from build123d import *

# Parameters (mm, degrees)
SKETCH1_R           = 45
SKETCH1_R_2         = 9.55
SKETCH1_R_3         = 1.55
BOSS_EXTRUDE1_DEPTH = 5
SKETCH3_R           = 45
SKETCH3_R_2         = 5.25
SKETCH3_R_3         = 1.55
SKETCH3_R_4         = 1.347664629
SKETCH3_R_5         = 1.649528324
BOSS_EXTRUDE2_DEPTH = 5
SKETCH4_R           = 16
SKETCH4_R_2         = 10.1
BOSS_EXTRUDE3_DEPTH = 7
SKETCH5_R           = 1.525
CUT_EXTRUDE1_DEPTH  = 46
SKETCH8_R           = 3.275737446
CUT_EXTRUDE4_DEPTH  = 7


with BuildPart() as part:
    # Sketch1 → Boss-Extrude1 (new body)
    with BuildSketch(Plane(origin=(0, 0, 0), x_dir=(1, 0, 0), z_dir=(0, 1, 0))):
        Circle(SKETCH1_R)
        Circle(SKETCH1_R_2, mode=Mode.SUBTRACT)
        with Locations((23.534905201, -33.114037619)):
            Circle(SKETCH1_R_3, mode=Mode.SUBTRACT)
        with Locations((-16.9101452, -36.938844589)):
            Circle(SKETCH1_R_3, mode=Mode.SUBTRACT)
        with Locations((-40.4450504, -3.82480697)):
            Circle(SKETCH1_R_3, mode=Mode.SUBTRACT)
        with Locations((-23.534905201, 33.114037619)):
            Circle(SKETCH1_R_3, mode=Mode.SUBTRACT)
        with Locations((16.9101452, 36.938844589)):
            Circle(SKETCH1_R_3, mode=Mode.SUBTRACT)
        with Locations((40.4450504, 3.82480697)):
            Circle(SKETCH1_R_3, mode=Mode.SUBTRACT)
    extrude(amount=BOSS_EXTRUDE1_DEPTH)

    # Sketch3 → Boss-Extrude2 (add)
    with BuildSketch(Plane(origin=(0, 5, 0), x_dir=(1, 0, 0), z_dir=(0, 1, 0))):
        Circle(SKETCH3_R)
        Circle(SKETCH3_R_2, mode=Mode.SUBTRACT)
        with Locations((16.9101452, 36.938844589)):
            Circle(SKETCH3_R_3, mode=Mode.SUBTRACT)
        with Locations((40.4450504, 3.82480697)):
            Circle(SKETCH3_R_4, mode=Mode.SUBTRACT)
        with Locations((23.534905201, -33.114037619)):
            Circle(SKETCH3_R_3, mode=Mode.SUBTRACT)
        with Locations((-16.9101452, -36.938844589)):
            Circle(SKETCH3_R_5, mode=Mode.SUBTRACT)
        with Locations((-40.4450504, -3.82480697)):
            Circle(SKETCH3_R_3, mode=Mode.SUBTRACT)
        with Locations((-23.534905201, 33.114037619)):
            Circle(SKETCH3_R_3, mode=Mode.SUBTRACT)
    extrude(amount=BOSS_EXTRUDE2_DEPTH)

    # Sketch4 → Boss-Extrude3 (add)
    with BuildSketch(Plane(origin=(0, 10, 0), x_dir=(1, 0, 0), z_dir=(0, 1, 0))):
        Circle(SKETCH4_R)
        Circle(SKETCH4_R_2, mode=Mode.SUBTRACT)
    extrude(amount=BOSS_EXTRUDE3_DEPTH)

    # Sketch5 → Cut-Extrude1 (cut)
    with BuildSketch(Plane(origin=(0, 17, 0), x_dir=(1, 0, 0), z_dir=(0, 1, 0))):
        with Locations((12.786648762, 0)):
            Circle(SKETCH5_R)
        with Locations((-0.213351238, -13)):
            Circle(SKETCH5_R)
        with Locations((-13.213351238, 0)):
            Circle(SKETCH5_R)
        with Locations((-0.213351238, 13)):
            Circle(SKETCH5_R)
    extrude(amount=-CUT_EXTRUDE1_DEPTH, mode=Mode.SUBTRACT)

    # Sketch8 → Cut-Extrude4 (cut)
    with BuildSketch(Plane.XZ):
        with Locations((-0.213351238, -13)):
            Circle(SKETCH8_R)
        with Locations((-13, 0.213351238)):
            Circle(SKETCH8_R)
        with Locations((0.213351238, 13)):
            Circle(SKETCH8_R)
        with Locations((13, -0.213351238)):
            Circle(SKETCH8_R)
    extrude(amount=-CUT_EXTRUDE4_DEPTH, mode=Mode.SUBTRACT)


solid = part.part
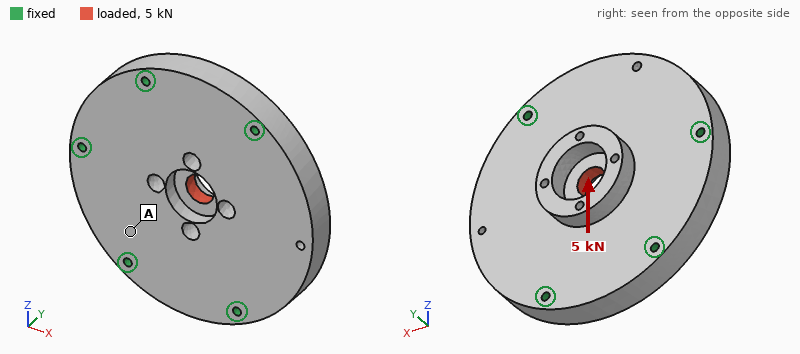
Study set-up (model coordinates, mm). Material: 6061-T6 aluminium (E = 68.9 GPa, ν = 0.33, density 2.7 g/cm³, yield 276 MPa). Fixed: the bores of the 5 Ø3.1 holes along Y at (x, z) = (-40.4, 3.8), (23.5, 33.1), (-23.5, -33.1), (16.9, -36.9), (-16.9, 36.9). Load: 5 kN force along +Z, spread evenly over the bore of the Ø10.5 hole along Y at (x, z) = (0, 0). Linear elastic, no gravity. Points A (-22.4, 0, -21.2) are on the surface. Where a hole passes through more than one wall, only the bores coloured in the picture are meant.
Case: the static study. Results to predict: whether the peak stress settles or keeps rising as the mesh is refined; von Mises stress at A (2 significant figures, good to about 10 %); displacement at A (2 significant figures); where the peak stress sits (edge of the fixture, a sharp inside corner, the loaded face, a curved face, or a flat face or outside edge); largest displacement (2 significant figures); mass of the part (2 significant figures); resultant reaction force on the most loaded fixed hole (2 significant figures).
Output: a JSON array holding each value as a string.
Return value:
["keeps rising", "5.4 MPa", "1.5 µm", "edge of the fixture", "7.8 µm", "170 g", "1.3 kN"]
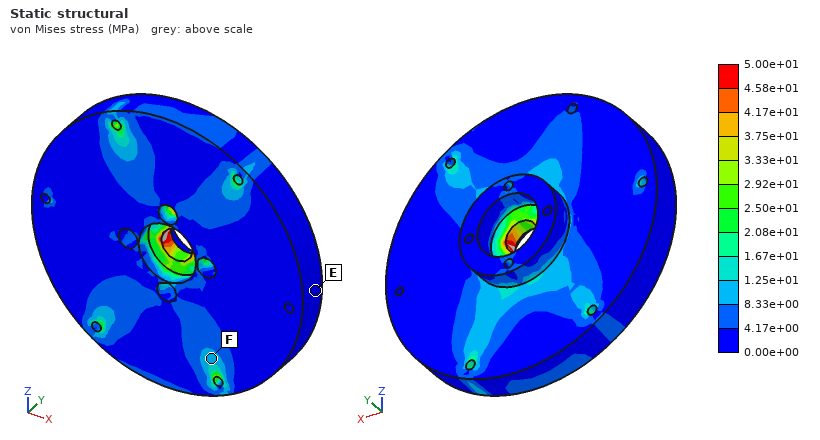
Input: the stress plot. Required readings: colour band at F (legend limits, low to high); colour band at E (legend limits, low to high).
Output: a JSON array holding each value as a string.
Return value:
["8.33e+00 to 1.25e+01 MPa", "0.00e+00 to 4.17e+00 MPa"]
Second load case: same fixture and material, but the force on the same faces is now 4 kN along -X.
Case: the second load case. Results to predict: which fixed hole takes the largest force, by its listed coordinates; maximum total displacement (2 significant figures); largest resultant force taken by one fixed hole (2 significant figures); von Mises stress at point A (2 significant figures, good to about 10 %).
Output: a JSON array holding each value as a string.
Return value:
["(-40.4, 3.8)", "7.4 µm", "1.2 kN", "3.1 MPa"]
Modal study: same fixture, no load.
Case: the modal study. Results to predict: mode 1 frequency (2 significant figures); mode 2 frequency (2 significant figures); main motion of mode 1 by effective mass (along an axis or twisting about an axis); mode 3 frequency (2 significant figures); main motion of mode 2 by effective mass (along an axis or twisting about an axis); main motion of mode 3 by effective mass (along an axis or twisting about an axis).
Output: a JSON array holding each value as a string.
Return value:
["6400 Hz", "9800 Hz", "along Y", "16 kHz", "along Y", "twisting about X"]
